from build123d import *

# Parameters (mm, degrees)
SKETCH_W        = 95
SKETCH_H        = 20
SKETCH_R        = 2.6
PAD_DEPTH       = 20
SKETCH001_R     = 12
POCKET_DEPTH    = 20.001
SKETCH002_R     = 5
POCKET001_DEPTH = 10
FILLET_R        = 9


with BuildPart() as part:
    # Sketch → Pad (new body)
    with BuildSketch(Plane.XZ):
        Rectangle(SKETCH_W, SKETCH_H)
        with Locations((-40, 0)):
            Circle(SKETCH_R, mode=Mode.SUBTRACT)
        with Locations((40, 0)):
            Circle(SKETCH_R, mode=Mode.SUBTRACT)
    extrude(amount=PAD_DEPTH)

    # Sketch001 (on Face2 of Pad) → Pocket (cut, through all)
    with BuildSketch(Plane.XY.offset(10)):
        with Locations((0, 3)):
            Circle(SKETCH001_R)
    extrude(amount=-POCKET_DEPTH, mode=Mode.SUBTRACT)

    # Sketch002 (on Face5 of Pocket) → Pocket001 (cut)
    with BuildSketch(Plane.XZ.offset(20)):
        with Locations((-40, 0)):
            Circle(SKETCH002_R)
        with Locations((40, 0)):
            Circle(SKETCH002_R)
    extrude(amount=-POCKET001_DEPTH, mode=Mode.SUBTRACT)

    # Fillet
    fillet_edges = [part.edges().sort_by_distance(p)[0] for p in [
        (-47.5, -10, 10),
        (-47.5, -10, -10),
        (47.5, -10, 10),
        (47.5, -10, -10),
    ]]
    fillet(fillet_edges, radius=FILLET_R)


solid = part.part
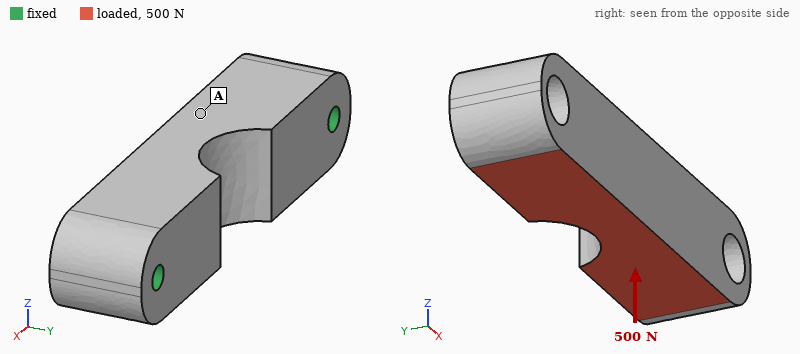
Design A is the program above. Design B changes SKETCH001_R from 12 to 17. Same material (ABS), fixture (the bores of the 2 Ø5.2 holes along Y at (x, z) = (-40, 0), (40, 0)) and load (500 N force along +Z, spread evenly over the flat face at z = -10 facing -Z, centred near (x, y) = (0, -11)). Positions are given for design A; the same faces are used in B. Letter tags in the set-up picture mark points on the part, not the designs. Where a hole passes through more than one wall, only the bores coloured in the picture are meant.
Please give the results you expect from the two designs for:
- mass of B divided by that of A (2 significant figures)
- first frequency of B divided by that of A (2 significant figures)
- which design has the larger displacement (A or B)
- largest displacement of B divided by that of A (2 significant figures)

0.87
1.0
B
1.2
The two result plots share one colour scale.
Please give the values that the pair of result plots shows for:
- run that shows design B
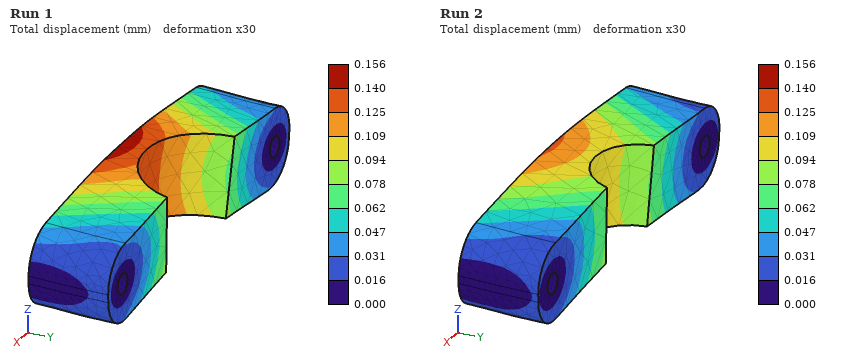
Run 1
